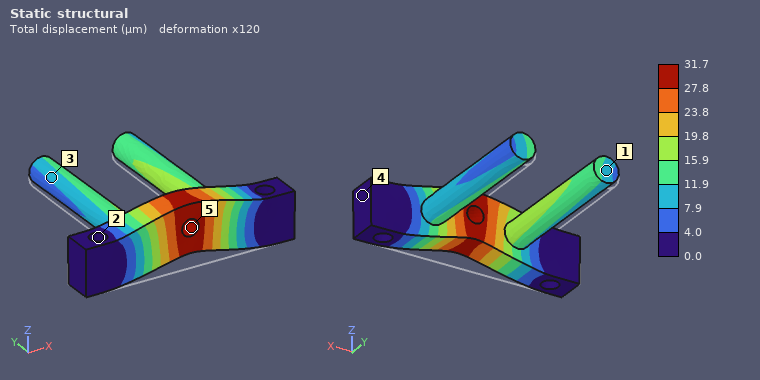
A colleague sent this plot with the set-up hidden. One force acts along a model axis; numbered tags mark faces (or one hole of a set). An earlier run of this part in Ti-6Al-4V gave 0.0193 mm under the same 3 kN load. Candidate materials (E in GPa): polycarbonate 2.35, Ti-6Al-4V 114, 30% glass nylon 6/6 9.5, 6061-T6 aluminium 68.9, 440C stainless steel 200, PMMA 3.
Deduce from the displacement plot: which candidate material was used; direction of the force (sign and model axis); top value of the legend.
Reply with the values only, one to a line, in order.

6061-T6 aluminium
+Z
31.7 µm
